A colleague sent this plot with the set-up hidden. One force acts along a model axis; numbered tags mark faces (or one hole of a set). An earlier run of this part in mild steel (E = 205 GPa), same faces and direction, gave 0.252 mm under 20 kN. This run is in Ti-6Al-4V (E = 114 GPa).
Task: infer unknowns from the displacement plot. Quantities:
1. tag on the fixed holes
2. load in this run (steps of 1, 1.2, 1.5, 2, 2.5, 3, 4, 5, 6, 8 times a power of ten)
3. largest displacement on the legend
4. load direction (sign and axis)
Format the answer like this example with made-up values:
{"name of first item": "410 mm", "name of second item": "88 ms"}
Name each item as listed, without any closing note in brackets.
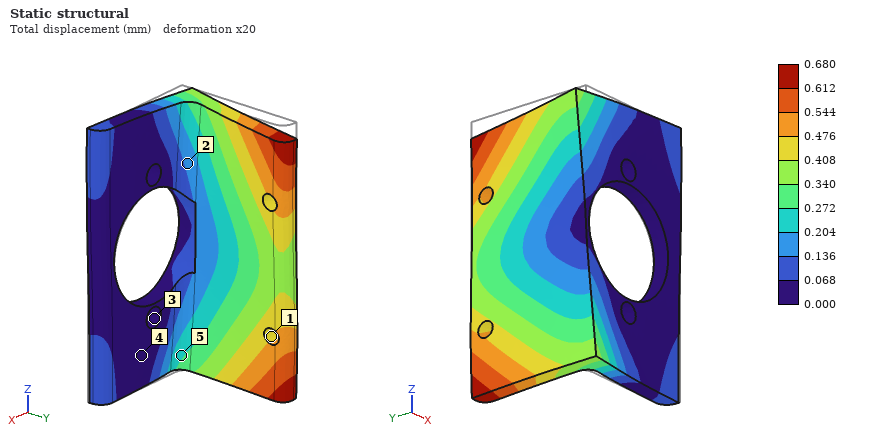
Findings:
{"tag on the fixed holes": "3", "load in this run": "30 kN", "largest displacement on the legend": "0.680 mm", "load direction": "-Z"}
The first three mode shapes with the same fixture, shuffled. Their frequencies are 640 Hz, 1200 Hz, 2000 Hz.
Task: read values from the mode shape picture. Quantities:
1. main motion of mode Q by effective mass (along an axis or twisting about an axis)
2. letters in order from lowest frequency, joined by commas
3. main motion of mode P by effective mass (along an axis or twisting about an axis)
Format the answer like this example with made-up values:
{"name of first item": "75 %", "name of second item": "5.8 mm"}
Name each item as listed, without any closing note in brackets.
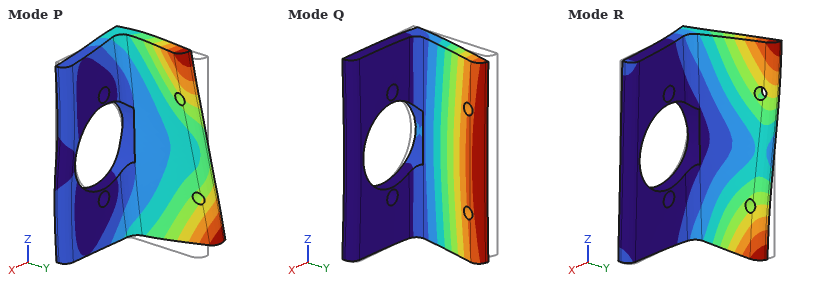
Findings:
{"main motion of mode Q by effective mass": "along X", "letters in order from lowest frequency, joined by commas": "Q, R, P", "main motion of mode P by effective mass": "along Z"}
